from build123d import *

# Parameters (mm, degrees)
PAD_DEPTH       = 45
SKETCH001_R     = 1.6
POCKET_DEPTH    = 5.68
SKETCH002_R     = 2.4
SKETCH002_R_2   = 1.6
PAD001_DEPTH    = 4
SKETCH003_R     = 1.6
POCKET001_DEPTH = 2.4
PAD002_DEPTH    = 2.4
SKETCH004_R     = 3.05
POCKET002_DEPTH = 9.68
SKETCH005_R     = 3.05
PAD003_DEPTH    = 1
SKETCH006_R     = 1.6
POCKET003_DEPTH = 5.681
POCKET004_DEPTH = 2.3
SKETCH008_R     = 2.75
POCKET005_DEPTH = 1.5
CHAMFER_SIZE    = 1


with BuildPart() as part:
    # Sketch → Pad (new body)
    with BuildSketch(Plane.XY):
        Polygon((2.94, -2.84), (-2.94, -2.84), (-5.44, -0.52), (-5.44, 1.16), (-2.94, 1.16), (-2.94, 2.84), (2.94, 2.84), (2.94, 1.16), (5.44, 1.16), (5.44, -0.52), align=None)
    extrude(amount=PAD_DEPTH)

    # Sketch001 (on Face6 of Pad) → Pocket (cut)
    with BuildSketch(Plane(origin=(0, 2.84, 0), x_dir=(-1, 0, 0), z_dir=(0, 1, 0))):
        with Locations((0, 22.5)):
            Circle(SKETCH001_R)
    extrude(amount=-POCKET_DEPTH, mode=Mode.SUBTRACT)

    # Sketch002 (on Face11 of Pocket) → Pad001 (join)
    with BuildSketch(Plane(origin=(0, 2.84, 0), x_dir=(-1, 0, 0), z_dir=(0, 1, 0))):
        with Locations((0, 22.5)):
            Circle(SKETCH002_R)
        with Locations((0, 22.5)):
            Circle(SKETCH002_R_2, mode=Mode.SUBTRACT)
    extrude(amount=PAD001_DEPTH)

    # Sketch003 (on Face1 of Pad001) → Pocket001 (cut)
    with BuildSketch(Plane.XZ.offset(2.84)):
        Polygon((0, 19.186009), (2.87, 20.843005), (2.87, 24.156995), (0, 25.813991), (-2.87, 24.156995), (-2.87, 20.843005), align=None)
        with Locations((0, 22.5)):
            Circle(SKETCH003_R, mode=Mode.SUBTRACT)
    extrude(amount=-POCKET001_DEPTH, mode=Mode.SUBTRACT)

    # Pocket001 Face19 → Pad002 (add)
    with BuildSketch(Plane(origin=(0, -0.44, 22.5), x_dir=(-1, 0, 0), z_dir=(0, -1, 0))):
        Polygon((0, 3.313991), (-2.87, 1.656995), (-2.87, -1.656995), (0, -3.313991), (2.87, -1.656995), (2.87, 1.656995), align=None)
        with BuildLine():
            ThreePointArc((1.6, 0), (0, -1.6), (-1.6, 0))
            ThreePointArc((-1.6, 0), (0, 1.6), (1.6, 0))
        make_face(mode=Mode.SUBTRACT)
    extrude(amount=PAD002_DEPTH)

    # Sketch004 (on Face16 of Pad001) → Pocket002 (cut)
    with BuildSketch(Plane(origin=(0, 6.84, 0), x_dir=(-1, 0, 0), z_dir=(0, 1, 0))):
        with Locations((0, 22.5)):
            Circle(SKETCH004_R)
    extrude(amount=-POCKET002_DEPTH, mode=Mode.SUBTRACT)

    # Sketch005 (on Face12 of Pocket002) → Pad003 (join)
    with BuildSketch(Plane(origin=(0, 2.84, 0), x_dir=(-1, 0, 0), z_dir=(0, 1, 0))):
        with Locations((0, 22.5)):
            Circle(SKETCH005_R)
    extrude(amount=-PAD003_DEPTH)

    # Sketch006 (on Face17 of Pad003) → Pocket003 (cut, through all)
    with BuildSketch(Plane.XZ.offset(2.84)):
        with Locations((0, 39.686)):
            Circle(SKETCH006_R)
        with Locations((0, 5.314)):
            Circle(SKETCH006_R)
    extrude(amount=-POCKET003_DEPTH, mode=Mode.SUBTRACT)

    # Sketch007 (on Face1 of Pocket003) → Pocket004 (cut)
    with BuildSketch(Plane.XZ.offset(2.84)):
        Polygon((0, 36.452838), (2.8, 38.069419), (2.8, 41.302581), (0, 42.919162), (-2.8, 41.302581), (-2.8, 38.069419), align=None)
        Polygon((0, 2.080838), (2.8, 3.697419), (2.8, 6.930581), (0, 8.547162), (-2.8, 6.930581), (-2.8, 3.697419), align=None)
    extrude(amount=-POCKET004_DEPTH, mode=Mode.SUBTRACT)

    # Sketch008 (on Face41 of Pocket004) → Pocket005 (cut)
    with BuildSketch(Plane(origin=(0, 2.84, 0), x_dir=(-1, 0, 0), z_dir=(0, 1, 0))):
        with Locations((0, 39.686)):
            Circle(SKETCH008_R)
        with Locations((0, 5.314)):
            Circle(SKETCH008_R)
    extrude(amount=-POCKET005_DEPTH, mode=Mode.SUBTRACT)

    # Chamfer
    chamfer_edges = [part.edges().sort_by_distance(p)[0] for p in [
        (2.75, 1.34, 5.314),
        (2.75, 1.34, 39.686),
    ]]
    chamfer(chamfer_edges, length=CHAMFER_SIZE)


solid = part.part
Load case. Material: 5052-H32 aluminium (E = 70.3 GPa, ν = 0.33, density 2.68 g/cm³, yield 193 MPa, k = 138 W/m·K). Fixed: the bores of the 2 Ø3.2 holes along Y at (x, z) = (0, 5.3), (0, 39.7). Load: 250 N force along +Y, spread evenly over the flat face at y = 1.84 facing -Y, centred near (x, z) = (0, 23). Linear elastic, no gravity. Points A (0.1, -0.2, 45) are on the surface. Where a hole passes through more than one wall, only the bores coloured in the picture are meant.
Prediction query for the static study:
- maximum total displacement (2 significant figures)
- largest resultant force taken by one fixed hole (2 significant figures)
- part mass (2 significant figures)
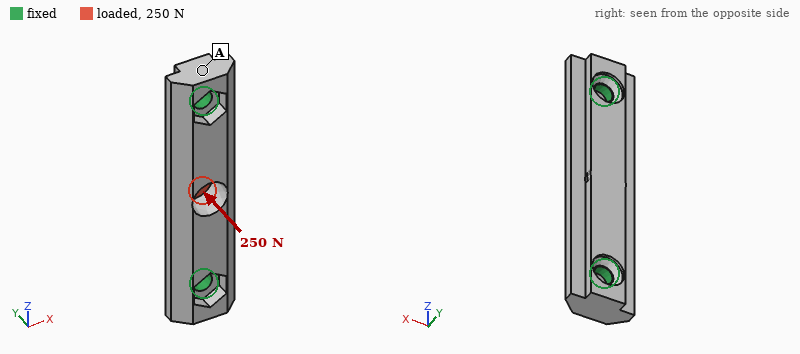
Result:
26 µm
130 N
4.8 g
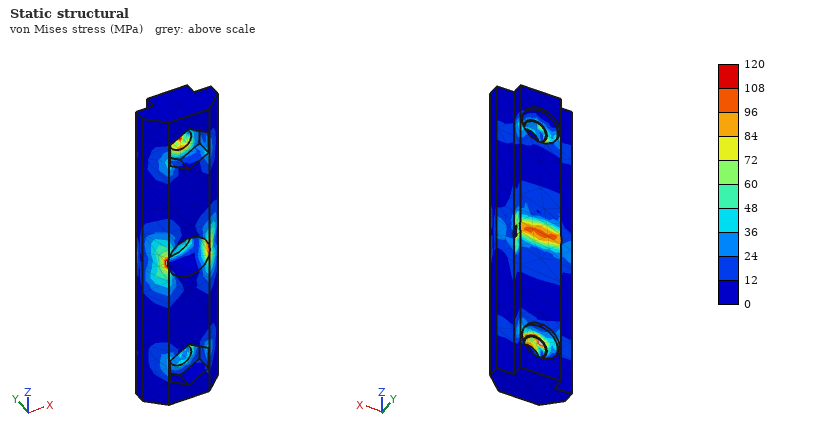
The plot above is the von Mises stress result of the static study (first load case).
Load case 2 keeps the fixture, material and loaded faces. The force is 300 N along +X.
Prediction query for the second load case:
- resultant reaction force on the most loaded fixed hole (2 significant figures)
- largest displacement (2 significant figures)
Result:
150 N
13 µm
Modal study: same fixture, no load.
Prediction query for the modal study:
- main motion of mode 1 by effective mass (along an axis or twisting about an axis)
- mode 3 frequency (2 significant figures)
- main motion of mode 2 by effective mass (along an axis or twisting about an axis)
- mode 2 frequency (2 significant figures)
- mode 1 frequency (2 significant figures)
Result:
along Y
26 kHz
along X
23 kHz
14 kHz
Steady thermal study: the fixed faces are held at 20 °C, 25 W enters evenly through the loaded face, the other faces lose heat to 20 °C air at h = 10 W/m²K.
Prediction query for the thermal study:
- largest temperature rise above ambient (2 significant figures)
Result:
64 K
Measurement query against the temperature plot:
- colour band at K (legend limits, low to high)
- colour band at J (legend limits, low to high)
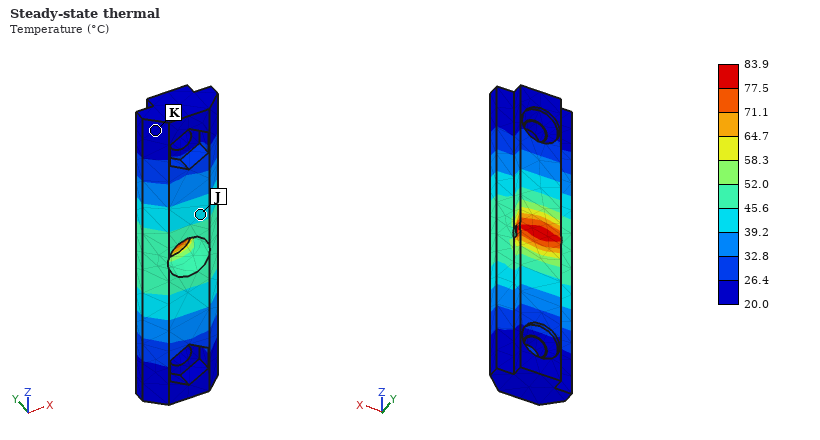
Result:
20.0 to 26.4 °C
39.2 to 45.6 °C
